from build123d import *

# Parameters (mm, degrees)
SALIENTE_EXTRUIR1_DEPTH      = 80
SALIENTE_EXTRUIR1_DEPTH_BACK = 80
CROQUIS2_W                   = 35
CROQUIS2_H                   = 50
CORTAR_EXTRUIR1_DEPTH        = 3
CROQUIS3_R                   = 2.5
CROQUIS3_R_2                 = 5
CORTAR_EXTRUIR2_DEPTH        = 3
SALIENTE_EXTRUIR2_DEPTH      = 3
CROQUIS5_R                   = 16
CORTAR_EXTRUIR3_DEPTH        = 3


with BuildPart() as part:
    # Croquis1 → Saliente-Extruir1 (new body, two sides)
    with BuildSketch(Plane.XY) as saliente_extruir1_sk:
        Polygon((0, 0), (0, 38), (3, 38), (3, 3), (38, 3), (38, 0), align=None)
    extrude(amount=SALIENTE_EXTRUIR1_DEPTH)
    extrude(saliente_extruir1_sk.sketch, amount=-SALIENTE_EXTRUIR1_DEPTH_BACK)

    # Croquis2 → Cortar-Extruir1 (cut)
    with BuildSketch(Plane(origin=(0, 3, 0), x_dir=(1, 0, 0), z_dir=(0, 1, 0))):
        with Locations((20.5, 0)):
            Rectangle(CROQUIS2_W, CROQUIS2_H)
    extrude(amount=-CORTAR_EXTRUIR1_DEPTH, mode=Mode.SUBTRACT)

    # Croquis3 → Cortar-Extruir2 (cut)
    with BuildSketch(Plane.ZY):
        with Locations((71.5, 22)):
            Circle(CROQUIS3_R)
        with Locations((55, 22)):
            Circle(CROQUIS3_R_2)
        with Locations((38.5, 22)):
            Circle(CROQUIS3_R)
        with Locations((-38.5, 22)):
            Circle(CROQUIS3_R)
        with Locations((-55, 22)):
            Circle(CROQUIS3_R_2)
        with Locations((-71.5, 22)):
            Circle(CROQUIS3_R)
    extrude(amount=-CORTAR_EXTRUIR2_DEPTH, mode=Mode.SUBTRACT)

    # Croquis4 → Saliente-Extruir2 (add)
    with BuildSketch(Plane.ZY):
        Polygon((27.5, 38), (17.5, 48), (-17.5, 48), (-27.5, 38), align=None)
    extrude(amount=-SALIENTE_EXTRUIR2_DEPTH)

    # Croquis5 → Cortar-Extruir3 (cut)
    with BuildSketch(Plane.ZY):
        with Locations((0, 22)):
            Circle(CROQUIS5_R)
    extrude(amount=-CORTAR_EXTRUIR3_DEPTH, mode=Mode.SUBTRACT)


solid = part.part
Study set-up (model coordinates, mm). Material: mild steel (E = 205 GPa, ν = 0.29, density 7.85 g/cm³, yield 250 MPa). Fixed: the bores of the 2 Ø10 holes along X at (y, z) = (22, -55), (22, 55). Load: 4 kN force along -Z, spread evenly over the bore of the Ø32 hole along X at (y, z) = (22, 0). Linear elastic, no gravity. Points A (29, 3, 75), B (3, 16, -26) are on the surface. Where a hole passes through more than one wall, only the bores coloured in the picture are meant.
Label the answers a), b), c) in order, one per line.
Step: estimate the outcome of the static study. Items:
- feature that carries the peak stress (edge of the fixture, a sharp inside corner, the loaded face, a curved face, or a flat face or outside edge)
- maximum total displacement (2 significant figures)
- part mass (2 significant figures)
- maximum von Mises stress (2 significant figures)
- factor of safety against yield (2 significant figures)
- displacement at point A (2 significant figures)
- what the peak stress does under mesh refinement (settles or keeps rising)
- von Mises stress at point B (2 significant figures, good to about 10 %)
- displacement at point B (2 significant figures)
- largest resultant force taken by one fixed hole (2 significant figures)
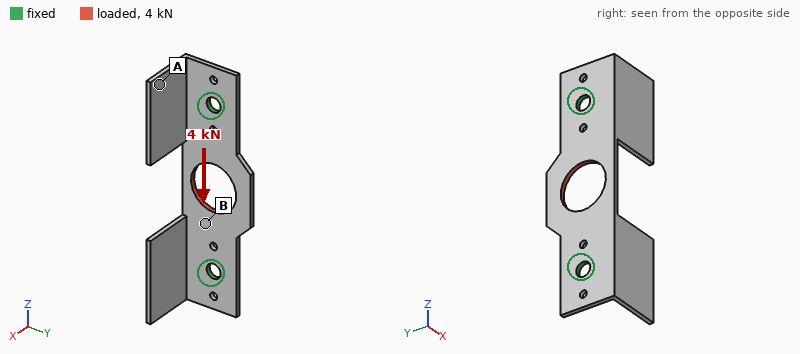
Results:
a) a curved face
b) 6.1 µm
c) 220 g
d) 67 MPa
e) 3.7
f) 2.8 µm
g) settles
h) 16 MPa
i) 3.1 µm
j) 2.0 kN
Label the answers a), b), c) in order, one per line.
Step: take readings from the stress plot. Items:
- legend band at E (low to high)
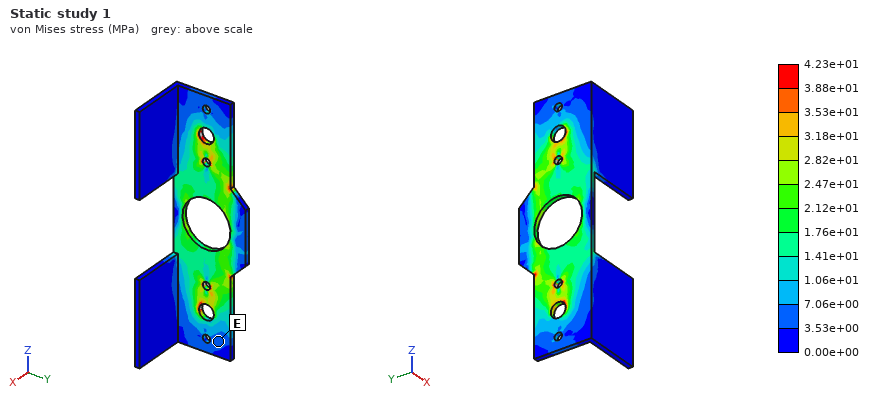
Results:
a) 3.53e+00 to 7.06e+00 MPa
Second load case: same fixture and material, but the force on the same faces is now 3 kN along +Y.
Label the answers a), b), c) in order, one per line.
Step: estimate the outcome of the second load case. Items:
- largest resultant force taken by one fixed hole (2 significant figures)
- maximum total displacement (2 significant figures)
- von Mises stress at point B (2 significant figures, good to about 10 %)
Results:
a) 1.5 kN
b) 22 µm
c) 25 MPa
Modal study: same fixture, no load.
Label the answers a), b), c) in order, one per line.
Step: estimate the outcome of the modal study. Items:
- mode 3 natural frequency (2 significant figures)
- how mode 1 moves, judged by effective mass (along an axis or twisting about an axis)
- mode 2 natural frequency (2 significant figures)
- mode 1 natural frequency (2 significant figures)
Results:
a) 1200 Hz
b) along Y
c) 1100 Hz
d) 1000 Hz
